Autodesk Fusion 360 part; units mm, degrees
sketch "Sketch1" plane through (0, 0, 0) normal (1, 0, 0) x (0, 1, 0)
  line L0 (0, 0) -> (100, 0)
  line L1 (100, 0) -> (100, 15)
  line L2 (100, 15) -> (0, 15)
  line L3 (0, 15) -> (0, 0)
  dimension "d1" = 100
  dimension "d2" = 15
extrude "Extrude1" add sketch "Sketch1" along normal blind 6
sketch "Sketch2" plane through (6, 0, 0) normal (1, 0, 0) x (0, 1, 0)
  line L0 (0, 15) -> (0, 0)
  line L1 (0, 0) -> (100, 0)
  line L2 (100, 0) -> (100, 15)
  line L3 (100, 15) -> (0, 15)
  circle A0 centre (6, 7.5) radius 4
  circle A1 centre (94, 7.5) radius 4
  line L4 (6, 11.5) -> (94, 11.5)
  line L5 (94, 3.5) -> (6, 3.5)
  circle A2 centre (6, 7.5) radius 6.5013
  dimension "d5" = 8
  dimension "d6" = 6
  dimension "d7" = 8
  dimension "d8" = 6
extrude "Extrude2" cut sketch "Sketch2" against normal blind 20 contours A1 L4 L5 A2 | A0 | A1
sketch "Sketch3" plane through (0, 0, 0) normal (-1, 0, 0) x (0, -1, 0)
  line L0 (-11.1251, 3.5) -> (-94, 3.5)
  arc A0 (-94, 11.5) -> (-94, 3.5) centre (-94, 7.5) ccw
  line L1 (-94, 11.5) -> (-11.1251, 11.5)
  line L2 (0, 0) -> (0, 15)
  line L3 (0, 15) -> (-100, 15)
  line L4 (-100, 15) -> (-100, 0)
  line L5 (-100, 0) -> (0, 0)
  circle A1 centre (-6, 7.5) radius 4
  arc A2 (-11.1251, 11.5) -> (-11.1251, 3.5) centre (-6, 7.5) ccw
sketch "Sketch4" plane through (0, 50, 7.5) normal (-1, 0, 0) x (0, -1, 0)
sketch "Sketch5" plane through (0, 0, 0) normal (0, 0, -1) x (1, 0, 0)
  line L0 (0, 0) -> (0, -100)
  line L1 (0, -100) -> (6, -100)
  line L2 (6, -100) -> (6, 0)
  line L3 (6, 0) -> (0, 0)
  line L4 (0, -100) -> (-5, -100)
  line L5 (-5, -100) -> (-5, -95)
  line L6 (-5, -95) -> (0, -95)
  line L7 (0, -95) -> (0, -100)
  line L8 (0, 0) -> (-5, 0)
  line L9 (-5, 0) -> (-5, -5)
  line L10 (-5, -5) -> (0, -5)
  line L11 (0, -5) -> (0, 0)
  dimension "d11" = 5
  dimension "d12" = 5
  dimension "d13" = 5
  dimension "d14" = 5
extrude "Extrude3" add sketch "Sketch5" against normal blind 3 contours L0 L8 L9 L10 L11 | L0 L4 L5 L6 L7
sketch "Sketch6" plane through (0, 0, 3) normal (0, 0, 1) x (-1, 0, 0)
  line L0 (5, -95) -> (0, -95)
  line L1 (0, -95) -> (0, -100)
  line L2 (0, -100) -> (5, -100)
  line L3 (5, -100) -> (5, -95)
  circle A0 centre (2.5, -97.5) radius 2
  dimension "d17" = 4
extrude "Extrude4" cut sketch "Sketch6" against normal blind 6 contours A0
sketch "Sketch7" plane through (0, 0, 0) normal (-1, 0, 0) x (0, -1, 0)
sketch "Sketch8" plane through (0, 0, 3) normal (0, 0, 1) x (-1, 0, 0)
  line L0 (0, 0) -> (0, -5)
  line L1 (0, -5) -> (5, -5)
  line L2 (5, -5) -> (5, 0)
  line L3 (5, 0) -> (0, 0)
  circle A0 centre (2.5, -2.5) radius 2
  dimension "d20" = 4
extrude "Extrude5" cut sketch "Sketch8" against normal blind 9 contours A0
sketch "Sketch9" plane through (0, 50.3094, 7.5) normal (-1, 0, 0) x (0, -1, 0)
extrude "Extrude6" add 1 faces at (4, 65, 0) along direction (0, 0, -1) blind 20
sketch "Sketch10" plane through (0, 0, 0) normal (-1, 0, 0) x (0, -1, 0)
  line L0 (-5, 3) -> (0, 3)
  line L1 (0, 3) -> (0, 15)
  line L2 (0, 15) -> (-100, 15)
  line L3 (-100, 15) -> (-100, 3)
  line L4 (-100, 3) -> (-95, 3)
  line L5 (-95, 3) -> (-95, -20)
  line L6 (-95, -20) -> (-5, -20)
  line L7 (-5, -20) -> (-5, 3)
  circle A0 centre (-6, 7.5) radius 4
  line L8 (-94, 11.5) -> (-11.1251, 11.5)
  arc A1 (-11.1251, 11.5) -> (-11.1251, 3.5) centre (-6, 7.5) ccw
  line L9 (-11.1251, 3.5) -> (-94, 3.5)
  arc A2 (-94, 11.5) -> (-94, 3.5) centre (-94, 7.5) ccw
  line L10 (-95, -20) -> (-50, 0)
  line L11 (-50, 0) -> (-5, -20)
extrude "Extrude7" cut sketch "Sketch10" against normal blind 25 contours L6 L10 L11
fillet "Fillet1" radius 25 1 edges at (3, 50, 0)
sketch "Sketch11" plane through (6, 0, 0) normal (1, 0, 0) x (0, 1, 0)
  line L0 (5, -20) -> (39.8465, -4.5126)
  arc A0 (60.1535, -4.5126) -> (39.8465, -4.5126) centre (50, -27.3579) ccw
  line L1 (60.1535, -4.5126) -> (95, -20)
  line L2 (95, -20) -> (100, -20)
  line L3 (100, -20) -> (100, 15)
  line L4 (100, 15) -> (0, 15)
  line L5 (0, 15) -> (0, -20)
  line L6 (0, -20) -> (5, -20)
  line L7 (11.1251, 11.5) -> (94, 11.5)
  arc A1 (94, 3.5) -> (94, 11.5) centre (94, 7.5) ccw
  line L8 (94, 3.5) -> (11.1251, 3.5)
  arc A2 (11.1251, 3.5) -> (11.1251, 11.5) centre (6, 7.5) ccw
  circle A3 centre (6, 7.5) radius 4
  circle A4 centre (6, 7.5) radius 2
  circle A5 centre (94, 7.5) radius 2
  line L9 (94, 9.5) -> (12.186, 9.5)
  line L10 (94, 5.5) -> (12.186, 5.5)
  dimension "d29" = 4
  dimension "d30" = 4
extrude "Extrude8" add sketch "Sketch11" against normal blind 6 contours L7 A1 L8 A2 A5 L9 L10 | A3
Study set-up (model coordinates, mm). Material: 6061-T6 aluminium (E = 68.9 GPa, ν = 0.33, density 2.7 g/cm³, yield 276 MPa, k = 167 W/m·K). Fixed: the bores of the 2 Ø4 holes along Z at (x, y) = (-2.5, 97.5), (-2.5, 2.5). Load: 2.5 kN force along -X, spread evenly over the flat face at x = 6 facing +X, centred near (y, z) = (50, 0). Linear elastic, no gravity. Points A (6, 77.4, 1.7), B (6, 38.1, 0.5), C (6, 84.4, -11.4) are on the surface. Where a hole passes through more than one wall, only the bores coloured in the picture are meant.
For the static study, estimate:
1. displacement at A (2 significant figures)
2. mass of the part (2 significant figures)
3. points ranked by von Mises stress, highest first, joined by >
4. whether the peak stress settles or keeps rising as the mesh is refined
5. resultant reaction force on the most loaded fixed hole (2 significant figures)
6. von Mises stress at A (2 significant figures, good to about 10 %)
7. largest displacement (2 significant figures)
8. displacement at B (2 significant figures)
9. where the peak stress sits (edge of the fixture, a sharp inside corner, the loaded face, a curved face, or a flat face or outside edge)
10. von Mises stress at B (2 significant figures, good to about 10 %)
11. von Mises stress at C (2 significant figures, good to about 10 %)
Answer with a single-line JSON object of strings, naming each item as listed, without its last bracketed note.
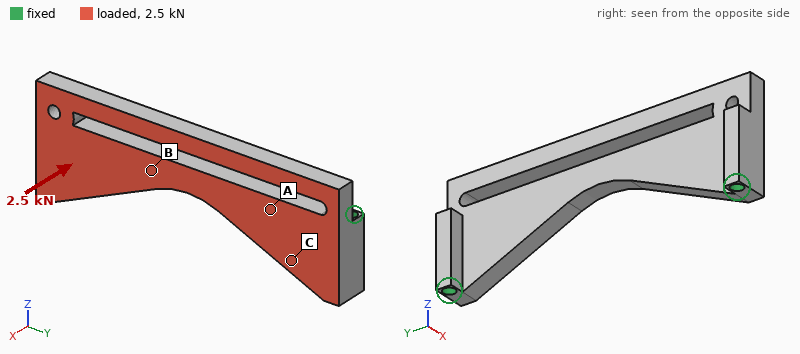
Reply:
{"displacement at A": "0.11 mm", "mass of the part": "38 g", "points ranked by von Mises stress, highest first, joined by >": "B > C > A", "whether the peak stress settles or keeps rising as the mesh is refined": "keeps rising", "resultant reaction force on the most loaded fixed hole": "1.6 kN", "von Mises stress at A": "16 MPa", "largest displacement": "0.38 mm", "displacement at B": "0.20 mm", "where the peak stress sits": "a sharp inside corner", "von Mises stress at B": "67 MPa", "von Mises stress at C": "38 MPa"}
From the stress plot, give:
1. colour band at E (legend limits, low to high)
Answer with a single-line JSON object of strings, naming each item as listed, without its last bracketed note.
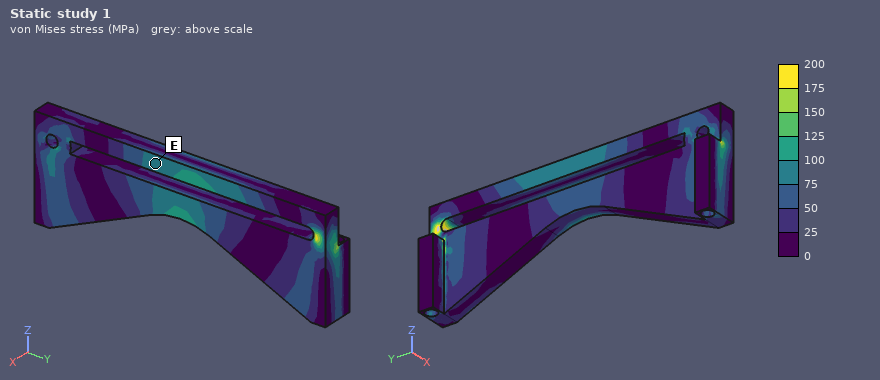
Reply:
{"colour band at E": "75 to 100 MPa"}
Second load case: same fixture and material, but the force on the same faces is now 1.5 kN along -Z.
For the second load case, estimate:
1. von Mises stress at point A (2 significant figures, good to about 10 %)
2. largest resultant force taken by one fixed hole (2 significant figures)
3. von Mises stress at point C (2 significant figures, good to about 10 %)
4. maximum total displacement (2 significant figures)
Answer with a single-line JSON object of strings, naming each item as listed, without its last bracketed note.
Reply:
{"von Mises stress at point A": "8.4 MPa", "largest resultant force taken by one fixed hole": "860 N", "von Mises stress at point C": "11 MPa", "maximum total displacement": "0.14 mm"}
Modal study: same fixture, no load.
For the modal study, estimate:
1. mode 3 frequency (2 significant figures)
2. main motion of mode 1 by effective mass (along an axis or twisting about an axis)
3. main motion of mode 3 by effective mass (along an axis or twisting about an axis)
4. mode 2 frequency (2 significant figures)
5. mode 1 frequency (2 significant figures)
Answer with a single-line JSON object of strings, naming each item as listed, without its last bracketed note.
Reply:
{"mode 3 frequency": "3700 Hz", "main motion of mode 1 by effective mass": "along X", "main motion of mode 3 by effective mass": "along X", "mode 2 frequency": "3200 Hz", "mode 1 frequency": "2600 Hz"}
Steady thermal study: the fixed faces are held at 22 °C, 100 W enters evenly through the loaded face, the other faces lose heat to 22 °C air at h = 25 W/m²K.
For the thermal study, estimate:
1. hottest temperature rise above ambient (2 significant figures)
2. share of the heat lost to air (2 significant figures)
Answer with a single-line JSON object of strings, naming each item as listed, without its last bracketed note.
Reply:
{"hottest temperature rise above ambient": "67 K", "share of the heat lost to air": "4.1 %"}
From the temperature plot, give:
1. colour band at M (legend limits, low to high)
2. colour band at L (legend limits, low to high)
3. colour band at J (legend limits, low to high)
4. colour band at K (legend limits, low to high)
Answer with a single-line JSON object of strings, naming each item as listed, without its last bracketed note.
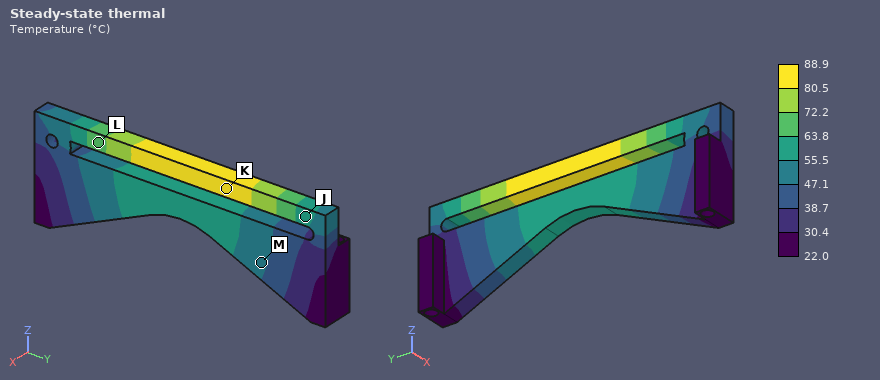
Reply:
{"colour band at M": "47.1 to 55.5 °C", "colour band at L": "63.8 to 72.2 °C", "colour band at J": "55.5 to 63.8 °C", "colour band at K": "80.5 to 88.9 °C"}
